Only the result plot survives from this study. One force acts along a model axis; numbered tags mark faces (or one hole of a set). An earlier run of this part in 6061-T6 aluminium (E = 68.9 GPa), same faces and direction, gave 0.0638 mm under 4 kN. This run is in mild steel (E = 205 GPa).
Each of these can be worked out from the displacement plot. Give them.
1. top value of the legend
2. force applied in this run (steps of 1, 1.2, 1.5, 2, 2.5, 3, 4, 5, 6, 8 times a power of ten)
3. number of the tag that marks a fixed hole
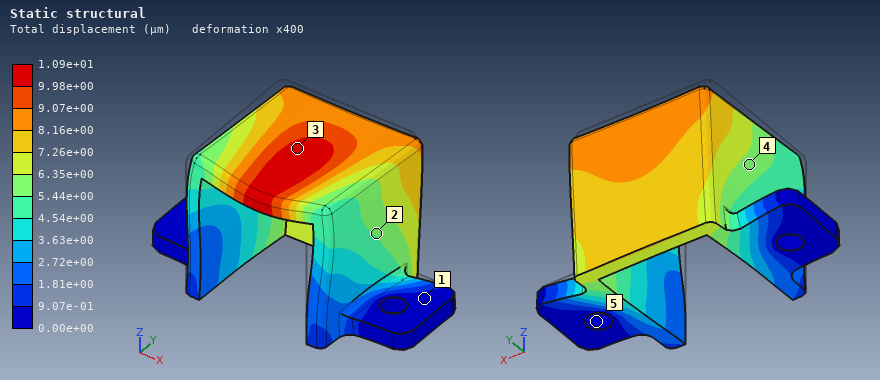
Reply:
1.09e+01 µm
2 kN
5
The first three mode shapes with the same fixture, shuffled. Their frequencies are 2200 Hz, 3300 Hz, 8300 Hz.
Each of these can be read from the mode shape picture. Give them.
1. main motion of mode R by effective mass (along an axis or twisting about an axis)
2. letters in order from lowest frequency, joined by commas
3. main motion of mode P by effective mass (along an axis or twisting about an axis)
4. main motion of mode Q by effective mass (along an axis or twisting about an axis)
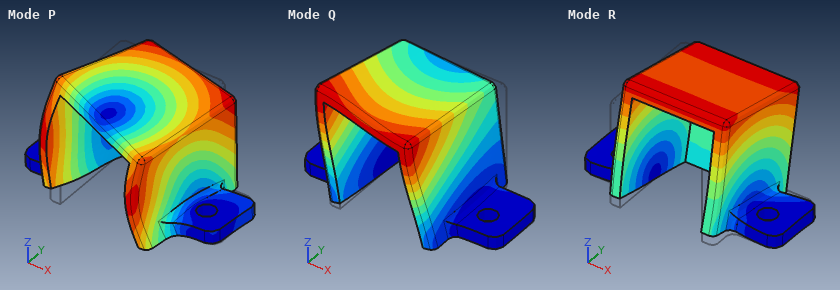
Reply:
along Y
R, Q, P
along X
along X
